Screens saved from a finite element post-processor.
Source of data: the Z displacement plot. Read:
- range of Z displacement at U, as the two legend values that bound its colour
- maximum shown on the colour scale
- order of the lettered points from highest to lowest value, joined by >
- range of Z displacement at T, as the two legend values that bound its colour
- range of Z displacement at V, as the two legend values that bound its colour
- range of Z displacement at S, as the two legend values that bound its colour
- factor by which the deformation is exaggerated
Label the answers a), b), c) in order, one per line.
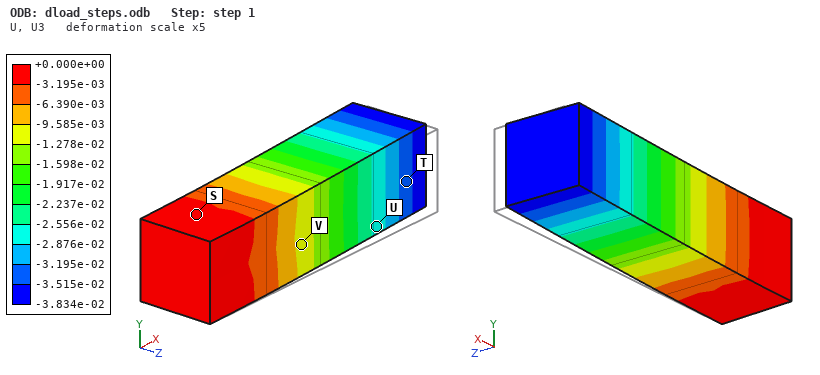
a) -2.876e-02 to -2.556e-02
b) +0.000e+00
c) S > V > U > T
d) -3.515e-02 to -3.195e-02
e) -1.278e-02 to -9.585e-03
f) -3.195e-03 to +0.000e+00
g) 5
